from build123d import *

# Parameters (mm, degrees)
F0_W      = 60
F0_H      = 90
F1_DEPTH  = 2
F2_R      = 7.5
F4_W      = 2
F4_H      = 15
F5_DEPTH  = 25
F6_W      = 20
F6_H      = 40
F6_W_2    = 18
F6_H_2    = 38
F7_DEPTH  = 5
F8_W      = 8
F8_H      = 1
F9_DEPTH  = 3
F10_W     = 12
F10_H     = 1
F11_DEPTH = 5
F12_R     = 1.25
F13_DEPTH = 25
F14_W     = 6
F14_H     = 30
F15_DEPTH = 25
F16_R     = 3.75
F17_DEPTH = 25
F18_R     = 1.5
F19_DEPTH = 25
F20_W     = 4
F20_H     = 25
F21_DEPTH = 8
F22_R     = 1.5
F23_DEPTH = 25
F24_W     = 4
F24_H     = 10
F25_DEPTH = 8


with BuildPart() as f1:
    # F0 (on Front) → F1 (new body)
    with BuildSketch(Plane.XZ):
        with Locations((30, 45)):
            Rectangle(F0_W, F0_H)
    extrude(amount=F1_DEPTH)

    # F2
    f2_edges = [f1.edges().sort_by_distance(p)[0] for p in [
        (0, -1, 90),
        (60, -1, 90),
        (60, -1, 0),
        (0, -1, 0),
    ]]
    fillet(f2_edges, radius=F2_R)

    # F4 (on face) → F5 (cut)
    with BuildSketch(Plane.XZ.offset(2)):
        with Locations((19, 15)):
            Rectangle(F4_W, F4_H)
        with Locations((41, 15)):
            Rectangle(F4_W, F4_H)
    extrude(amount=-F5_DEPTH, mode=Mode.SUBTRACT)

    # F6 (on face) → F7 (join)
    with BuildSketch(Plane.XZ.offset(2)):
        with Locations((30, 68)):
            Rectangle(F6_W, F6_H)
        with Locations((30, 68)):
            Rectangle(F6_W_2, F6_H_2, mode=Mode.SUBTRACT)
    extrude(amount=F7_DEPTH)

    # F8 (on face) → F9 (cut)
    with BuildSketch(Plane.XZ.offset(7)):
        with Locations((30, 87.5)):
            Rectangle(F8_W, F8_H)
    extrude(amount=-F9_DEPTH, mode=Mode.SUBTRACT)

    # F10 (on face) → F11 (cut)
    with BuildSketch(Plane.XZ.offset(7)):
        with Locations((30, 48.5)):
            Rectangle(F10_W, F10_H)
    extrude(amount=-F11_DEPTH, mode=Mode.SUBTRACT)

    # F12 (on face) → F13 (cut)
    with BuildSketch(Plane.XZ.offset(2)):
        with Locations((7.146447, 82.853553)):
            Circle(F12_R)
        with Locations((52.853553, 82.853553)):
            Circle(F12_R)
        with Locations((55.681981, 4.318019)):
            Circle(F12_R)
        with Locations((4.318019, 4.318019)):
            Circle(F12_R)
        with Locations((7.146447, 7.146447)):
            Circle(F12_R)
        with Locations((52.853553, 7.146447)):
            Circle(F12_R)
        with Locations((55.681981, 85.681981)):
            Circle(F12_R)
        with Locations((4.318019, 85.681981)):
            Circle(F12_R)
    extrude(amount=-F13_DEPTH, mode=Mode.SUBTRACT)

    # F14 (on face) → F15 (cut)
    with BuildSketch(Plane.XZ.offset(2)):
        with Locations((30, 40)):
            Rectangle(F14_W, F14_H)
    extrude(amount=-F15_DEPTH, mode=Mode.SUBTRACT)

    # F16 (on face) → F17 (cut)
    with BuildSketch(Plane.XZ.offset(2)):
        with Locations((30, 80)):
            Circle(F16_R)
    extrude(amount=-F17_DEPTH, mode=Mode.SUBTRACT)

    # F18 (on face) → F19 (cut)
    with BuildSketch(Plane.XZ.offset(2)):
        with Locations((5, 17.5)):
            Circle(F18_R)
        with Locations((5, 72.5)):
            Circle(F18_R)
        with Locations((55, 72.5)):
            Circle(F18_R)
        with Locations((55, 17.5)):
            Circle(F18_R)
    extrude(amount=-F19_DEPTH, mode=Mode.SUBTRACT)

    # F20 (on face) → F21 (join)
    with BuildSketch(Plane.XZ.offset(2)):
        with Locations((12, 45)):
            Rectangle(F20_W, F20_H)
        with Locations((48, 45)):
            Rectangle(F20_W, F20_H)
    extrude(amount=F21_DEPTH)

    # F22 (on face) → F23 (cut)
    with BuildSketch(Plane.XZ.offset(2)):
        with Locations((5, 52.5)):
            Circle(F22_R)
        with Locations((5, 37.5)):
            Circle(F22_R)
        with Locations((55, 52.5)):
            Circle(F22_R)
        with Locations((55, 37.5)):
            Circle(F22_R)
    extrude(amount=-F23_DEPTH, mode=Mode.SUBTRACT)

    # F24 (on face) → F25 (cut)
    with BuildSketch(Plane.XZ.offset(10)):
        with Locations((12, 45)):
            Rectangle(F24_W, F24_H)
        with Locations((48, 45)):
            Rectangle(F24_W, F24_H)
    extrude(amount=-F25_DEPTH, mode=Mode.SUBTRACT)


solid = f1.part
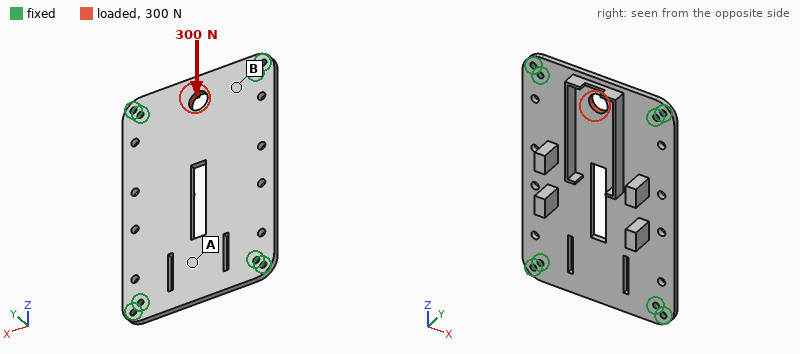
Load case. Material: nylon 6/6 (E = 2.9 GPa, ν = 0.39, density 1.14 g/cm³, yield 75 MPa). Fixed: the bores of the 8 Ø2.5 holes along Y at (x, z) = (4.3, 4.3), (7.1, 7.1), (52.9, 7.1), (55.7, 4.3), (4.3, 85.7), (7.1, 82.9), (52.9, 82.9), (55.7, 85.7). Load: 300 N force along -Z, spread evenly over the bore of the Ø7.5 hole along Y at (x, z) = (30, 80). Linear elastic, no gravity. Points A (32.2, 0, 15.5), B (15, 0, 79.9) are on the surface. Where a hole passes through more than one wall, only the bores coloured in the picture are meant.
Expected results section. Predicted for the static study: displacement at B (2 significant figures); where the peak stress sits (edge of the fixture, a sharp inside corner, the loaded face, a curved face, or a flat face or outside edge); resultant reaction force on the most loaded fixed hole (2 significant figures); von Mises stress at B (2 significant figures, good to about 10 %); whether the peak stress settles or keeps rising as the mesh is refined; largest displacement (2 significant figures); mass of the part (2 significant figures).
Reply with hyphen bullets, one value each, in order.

- 30 µm
- edge of the fixture
- 90 N
- 3.7 MPa
- keeps rising
- 89 µm
- 13 g
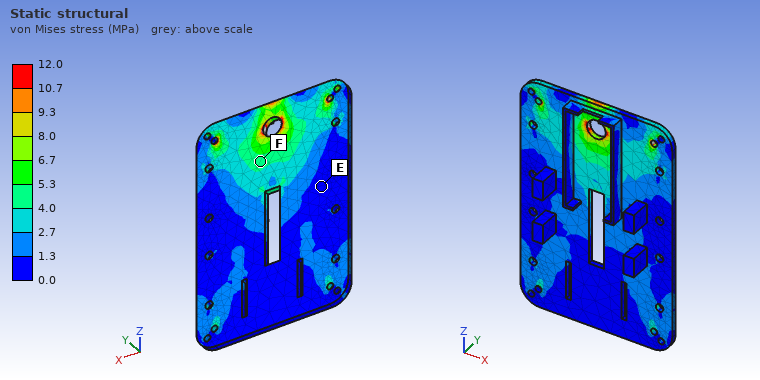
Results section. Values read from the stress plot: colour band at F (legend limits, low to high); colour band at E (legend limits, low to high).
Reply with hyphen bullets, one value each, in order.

- 4.0 to 5.3 MPa
- 0.0 to 1.3 MPa
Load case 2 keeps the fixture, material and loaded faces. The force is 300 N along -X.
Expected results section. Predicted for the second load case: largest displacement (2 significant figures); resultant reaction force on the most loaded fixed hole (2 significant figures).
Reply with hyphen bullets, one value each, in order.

- 43 µm
- 100 N
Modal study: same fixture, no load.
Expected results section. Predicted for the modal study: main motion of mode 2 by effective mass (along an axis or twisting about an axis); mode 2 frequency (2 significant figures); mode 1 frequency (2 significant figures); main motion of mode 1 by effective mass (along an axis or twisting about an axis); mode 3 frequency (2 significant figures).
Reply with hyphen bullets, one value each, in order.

- twisting about Z
- 660 Hz
- 470 Hz
- along Y
- 1000 Hz
